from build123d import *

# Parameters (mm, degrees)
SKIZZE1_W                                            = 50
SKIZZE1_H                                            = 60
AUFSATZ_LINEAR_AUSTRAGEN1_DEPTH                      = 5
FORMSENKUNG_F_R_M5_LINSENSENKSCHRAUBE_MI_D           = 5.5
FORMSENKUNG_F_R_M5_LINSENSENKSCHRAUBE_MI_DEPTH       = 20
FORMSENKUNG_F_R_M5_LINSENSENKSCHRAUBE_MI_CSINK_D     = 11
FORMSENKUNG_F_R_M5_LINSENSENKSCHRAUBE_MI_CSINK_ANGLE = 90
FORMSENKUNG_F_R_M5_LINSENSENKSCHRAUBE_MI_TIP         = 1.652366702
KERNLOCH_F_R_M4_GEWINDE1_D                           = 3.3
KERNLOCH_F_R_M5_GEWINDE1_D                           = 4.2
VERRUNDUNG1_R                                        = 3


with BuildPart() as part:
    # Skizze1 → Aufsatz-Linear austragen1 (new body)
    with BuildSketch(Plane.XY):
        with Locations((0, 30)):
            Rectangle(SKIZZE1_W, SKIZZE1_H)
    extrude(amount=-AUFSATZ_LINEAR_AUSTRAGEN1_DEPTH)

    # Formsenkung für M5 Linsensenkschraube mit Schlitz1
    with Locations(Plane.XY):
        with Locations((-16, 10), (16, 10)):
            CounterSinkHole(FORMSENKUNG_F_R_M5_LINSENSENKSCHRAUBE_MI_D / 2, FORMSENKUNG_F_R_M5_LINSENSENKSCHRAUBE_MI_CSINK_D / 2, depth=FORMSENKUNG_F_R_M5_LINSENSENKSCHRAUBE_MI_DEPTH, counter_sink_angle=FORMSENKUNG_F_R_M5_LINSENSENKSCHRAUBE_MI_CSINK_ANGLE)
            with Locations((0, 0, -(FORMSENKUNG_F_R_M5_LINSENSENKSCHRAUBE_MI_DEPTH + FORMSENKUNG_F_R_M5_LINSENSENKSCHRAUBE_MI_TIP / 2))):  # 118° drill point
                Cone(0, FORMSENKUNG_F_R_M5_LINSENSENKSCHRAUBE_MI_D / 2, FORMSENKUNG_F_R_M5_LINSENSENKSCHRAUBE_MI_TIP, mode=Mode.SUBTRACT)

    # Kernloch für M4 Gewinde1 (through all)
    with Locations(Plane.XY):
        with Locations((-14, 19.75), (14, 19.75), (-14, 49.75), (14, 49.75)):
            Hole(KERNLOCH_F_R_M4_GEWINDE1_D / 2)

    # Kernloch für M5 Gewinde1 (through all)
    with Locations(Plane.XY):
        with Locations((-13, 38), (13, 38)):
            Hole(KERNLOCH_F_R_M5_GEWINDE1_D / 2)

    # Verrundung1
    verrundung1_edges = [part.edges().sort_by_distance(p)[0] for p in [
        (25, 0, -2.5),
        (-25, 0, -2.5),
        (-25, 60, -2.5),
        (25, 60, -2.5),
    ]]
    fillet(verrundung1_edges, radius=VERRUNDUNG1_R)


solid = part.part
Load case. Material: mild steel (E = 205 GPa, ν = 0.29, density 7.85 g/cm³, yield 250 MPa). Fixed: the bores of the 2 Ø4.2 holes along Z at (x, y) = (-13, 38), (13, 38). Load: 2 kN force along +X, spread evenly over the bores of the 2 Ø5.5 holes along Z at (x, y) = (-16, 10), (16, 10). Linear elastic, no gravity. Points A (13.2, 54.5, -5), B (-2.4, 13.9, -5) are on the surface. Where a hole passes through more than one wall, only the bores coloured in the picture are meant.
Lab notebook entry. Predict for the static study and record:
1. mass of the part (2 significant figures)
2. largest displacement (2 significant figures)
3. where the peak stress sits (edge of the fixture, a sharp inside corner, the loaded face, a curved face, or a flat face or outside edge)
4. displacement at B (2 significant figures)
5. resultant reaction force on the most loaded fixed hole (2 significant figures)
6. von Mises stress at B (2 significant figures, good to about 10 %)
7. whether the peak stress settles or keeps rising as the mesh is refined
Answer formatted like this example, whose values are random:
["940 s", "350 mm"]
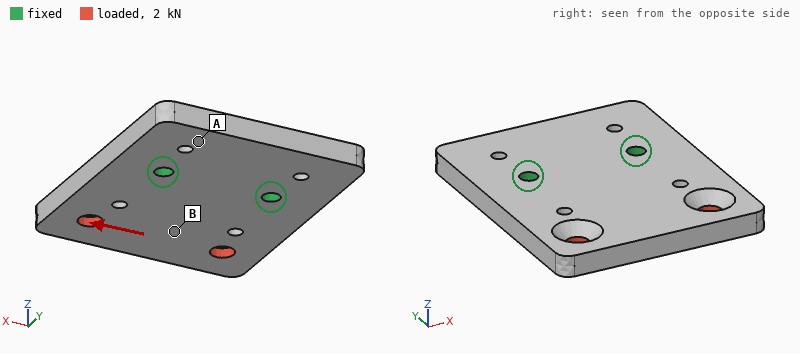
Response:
["110 g", "13 µm", "edge of the fixture", "5.8 µm", "2.2 kN", "23 MPa", "keeps rising"]
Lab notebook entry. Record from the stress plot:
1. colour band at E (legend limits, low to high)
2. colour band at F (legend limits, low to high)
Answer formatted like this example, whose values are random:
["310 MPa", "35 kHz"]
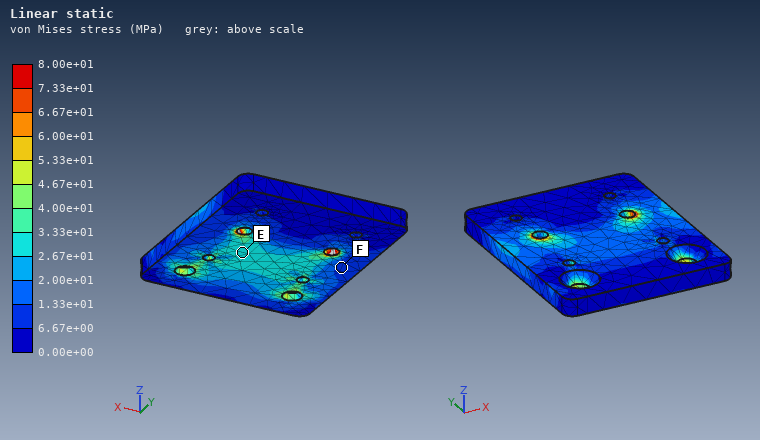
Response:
["2.67e+01 to 3.33e+01 MPa", "6.67e+00 to 1.33e+01 MPa"]
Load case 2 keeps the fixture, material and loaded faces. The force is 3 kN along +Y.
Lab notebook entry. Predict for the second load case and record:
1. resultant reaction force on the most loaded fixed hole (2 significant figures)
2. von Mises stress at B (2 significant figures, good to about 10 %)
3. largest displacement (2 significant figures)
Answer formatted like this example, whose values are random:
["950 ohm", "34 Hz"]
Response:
["1.5 kN", "19 MPa", "28 µm"]
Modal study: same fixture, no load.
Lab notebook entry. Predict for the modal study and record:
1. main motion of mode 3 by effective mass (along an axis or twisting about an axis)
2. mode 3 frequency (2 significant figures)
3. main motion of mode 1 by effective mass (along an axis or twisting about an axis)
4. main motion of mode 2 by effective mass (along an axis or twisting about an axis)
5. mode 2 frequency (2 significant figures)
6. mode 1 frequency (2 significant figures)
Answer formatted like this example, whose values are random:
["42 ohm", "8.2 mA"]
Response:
["along Z", "7800 Hz", "along Z", "twisting about Y", "5400 Hz", "2800 Hz"]
